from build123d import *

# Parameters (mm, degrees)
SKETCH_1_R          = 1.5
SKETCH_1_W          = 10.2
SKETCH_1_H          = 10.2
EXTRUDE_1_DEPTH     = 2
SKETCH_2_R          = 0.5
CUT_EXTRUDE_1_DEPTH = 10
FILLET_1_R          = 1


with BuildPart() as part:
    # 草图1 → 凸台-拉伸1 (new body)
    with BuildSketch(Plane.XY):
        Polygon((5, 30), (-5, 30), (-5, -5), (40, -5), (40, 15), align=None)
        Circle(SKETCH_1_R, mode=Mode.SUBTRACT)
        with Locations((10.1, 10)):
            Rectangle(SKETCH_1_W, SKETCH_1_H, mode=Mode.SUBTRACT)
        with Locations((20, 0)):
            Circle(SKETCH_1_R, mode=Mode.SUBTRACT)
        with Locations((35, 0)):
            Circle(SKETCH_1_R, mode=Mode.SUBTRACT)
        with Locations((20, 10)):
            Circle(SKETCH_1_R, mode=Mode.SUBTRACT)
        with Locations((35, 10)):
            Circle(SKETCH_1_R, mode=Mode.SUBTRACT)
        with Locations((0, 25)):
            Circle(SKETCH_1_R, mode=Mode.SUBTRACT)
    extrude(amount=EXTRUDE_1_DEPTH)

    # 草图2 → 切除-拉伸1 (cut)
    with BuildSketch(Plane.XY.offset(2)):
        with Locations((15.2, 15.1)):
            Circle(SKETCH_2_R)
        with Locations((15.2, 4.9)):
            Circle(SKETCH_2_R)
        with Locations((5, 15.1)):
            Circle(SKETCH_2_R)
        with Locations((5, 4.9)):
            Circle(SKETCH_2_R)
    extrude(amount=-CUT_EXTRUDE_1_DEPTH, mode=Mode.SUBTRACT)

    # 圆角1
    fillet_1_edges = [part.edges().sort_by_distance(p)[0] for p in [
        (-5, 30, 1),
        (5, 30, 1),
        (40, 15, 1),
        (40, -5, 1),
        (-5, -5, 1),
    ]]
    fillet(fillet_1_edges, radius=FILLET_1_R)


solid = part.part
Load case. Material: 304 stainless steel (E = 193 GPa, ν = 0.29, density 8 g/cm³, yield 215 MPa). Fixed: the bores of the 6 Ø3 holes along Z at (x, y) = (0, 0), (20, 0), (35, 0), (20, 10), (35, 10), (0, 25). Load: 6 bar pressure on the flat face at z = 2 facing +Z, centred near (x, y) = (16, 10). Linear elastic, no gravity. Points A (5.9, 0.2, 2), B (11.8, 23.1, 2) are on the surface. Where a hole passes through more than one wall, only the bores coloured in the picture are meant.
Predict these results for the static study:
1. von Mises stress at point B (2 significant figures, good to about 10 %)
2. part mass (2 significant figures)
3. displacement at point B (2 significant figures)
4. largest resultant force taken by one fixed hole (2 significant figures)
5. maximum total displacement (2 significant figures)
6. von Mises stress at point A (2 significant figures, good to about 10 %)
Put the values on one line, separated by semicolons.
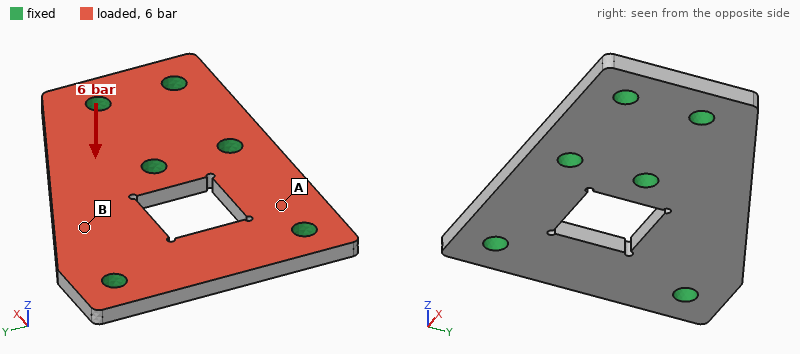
24 MPa; 19 g; 7.5 µm; 160 N; 11 µm; 11 MPa
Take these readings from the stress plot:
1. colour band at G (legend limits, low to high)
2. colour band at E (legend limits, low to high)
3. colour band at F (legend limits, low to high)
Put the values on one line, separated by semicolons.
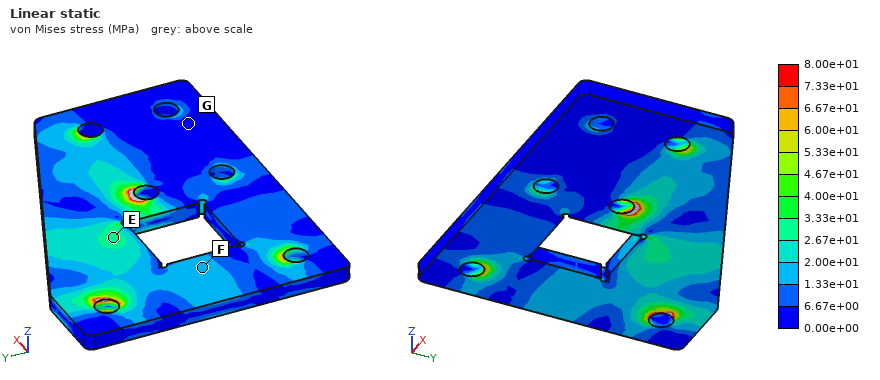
0.00e+00 to 6.67e+00 MPa; 2.67e+01 to 3.33e+01 MPa; 1.33e+01 to 2.00e+01 MPa
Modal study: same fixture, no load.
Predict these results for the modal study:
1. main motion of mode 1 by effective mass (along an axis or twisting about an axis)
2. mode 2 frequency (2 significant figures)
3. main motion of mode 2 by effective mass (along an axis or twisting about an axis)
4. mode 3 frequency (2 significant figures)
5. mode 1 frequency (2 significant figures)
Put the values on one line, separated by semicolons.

along Z; 17 kHz; along Z; 21 kHz; 12 kHz
